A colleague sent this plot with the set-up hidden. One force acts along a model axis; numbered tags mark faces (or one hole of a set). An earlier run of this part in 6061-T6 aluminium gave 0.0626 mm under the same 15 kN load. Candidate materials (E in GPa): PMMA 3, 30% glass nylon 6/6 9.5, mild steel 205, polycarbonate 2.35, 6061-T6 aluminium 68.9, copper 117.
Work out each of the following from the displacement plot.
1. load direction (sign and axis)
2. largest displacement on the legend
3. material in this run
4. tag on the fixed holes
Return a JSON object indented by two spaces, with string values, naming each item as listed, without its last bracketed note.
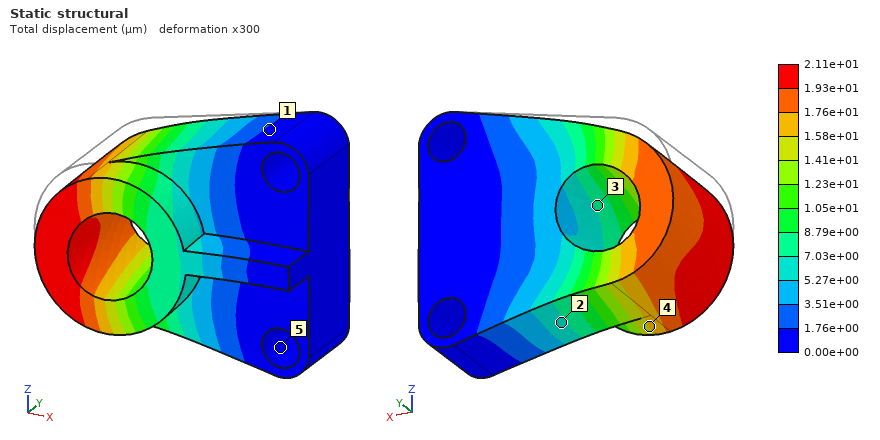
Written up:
{
  "load direction": "-Z",
  "largest displacement on the legend": "2.11e+01 µm",
  "material in this run": "mild steel",
  "tag on the fixed holes": "5"
}
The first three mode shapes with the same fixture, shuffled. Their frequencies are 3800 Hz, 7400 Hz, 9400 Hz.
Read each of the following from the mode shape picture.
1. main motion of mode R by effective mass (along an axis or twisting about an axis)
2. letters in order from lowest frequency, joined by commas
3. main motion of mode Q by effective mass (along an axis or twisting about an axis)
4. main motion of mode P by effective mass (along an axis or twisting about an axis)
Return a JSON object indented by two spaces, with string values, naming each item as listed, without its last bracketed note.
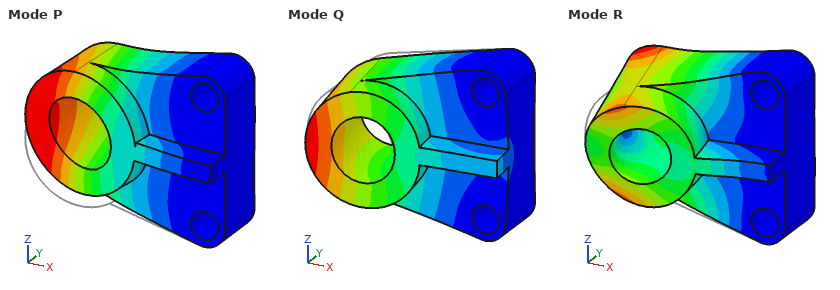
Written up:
{
  "main motion of mode R by effective mass": "twisting about X",
  "letters in order from lowest frequency, joined by commas": "Q, P, R",
  "main motion of mode Q by effective mass": "along Y",
  "main motion of mode P by effective mass": "along Z"
}
